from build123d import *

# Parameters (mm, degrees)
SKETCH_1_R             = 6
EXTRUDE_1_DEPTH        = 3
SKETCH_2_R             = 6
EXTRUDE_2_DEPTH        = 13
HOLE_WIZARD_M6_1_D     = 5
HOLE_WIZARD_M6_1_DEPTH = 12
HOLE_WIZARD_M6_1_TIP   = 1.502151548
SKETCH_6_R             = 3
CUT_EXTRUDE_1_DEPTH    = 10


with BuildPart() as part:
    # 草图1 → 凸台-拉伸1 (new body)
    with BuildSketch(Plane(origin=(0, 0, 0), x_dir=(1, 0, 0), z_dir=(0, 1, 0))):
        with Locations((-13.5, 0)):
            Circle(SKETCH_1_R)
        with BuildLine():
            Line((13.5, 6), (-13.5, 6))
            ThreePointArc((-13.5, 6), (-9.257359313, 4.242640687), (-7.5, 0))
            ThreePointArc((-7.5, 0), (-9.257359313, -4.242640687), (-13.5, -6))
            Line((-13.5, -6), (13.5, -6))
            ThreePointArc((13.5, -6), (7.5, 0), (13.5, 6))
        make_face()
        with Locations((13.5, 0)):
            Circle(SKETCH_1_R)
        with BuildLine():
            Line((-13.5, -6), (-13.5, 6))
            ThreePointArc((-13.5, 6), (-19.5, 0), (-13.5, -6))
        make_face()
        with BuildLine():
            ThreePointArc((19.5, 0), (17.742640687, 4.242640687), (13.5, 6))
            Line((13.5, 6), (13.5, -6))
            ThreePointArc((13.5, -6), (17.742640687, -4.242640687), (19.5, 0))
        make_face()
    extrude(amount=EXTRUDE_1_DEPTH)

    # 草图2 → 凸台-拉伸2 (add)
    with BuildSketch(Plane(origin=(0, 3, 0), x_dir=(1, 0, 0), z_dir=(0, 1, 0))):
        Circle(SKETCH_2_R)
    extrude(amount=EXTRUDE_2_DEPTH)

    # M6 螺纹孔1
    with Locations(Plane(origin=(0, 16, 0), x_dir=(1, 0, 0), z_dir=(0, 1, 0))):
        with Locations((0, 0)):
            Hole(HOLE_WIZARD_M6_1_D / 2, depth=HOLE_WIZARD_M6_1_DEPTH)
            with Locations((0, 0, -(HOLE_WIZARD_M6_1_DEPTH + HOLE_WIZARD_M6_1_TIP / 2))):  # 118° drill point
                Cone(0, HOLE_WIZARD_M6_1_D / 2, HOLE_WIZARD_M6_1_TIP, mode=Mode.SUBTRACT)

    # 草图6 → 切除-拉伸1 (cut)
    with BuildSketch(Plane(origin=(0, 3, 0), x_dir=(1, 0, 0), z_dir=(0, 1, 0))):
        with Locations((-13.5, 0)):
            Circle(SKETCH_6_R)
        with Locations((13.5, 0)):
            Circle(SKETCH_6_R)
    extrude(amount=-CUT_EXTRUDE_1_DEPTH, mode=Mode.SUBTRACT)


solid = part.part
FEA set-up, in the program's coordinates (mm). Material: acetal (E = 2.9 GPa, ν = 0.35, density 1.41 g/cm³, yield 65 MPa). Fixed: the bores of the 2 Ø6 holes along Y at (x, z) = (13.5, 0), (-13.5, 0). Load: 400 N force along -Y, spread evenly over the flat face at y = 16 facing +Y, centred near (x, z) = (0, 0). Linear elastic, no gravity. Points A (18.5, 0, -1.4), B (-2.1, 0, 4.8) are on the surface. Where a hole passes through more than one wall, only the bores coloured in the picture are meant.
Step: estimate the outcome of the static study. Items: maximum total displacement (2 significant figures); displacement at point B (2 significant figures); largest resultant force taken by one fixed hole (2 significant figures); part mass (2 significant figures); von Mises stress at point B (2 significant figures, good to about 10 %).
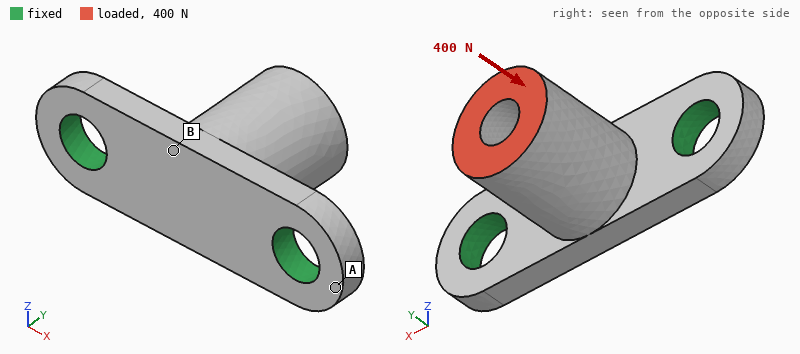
0.15 mm
0.14 mm
210 N
3.3 g
11 MPa
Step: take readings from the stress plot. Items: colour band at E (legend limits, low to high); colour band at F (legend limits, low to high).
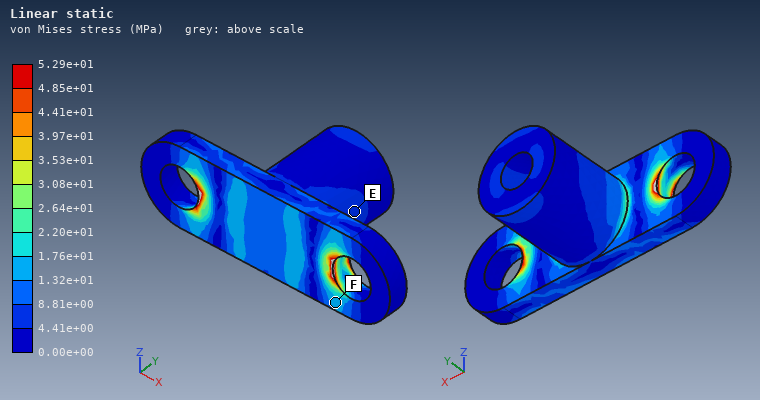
4.41e+00 to 8.81e+00 MPa
1.32e+01 to 1.76e+01 MPa
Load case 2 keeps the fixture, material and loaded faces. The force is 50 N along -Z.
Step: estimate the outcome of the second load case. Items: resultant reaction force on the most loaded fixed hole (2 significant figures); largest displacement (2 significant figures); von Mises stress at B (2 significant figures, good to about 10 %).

25 N
0.31 mm
7.0 MPa
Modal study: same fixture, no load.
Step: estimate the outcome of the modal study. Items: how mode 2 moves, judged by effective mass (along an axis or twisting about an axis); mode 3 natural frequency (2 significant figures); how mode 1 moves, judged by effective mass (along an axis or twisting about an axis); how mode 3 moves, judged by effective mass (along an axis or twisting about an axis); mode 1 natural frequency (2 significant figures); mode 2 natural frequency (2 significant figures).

along X
5500 Hz
along Z
along Y
2400 Hz
5200 Hz
